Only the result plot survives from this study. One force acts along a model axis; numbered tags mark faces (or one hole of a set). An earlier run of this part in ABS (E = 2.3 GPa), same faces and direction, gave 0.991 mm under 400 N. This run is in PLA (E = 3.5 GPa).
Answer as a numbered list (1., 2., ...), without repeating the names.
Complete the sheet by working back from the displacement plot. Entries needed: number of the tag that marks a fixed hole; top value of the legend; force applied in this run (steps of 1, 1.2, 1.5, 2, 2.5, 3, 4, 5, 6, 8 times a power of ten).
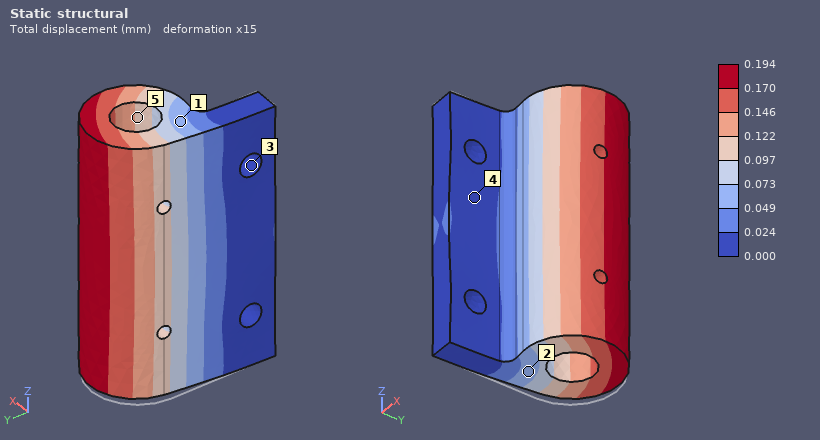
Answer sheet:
1. 3
2. 0.194 mm
3. 120 N
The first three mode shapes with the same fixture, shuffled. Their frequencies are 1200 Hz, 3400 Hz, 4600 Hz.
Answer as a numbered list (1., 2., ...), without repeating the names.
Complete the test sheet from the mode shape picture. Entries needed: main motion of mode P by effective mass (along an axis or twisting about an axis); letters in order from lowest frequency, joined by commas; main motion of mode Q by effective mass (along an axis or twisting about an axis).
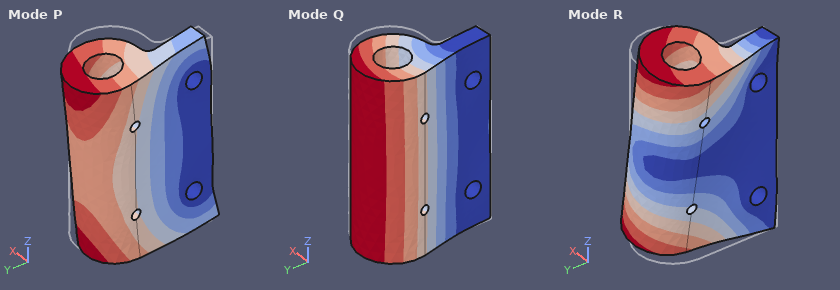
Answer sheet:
1. along Z
2. Q, R, P
3. along X
